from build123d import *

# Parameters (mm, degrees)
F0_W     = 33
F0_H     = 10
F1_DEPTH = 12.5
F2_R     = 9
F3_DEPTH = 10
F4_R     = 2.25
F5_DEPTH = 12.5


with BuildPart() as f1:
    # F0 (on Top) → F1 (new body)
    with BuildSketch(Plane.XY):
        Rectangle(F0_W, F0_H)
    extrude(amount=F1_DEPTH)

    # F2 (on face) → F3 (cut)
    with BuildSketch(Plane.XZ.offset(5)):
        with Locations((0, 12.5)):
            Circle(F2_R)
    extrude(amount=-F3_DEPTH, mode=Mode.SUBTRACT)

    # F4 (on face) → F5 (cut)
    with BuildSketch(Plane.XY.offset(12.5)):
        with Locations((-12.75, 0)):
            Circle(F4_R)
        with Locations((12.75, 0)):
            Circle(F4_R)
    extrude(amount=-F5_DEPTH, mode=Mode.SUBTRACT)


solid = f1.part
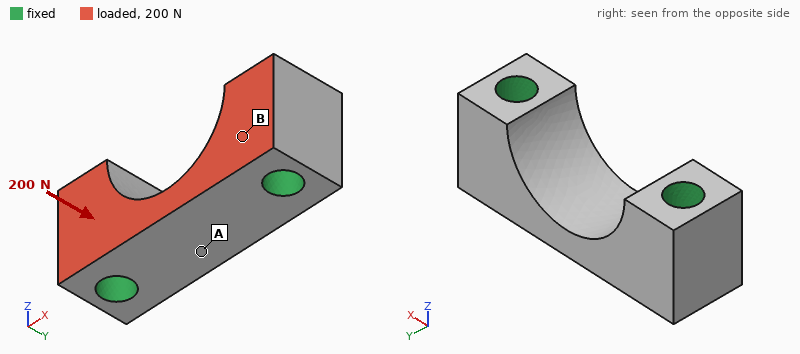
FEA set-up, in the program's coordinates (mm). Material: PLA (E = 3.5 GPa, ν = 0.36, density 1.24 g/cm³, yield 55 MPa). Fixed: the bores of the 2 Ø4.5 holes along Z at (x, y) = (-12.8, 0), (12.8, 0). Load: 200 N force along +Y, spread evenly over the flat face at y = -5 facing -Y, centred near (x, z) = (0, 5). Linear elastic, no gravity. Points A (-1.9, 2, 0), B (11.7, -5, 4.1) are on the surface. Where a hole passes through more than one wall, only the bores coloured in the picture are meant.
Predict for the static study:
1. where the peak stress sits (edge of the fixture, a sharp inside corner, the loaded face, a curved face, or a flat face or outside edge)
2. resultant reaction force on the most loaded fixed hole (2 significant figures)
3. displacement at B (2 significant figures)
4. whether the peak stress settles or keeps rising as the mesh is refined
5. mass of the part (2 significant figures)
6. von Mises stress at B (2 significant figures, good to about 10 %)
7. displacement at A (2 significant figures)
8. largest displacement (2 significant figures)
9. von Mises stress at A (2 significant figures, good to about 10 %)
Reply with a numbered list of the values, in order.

1. edge of the fixture
2. 100 N
3. 1.3 µm
4. keeps rising
5. 3.0 g
6. 1.4 MPa
7. 5.9 µm
8. 7.2 µm
9. 0.55 MPa
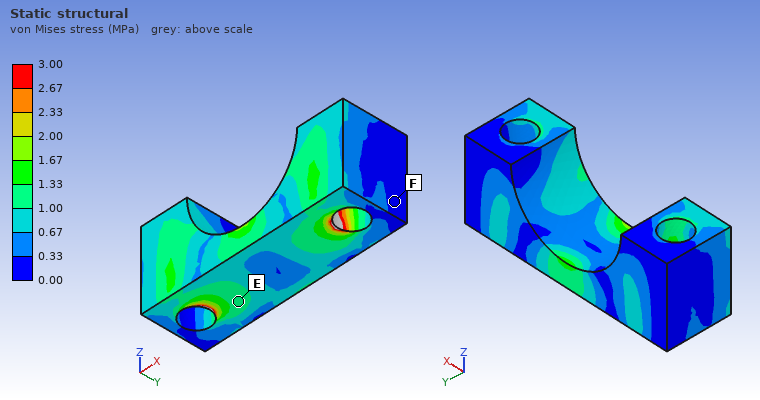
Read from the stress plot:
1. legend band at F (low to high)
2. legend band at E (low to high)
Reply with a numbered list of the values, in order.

1. 0.00 to 0.33 MPa
2. 1.00 to 1.33 MPa
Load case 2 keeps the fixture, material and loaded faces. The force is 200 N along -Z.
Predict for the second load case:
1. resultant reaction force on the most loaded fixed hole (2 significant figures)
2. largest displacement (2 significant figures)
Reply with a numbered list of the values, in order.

1. 100 N
2. 15 µm
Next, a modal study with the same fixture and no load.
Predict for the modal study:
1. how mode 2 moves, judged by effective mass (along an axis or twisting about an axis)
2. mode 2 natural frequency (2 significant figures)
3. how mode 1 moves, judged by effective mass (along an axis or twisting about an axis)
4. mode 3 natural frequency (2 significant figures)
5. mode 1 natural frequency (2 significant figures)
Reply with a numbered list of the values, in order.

1. along Z
2. 21 kHz
3. along Y
4. 28 kHz
5. 18 kHz
